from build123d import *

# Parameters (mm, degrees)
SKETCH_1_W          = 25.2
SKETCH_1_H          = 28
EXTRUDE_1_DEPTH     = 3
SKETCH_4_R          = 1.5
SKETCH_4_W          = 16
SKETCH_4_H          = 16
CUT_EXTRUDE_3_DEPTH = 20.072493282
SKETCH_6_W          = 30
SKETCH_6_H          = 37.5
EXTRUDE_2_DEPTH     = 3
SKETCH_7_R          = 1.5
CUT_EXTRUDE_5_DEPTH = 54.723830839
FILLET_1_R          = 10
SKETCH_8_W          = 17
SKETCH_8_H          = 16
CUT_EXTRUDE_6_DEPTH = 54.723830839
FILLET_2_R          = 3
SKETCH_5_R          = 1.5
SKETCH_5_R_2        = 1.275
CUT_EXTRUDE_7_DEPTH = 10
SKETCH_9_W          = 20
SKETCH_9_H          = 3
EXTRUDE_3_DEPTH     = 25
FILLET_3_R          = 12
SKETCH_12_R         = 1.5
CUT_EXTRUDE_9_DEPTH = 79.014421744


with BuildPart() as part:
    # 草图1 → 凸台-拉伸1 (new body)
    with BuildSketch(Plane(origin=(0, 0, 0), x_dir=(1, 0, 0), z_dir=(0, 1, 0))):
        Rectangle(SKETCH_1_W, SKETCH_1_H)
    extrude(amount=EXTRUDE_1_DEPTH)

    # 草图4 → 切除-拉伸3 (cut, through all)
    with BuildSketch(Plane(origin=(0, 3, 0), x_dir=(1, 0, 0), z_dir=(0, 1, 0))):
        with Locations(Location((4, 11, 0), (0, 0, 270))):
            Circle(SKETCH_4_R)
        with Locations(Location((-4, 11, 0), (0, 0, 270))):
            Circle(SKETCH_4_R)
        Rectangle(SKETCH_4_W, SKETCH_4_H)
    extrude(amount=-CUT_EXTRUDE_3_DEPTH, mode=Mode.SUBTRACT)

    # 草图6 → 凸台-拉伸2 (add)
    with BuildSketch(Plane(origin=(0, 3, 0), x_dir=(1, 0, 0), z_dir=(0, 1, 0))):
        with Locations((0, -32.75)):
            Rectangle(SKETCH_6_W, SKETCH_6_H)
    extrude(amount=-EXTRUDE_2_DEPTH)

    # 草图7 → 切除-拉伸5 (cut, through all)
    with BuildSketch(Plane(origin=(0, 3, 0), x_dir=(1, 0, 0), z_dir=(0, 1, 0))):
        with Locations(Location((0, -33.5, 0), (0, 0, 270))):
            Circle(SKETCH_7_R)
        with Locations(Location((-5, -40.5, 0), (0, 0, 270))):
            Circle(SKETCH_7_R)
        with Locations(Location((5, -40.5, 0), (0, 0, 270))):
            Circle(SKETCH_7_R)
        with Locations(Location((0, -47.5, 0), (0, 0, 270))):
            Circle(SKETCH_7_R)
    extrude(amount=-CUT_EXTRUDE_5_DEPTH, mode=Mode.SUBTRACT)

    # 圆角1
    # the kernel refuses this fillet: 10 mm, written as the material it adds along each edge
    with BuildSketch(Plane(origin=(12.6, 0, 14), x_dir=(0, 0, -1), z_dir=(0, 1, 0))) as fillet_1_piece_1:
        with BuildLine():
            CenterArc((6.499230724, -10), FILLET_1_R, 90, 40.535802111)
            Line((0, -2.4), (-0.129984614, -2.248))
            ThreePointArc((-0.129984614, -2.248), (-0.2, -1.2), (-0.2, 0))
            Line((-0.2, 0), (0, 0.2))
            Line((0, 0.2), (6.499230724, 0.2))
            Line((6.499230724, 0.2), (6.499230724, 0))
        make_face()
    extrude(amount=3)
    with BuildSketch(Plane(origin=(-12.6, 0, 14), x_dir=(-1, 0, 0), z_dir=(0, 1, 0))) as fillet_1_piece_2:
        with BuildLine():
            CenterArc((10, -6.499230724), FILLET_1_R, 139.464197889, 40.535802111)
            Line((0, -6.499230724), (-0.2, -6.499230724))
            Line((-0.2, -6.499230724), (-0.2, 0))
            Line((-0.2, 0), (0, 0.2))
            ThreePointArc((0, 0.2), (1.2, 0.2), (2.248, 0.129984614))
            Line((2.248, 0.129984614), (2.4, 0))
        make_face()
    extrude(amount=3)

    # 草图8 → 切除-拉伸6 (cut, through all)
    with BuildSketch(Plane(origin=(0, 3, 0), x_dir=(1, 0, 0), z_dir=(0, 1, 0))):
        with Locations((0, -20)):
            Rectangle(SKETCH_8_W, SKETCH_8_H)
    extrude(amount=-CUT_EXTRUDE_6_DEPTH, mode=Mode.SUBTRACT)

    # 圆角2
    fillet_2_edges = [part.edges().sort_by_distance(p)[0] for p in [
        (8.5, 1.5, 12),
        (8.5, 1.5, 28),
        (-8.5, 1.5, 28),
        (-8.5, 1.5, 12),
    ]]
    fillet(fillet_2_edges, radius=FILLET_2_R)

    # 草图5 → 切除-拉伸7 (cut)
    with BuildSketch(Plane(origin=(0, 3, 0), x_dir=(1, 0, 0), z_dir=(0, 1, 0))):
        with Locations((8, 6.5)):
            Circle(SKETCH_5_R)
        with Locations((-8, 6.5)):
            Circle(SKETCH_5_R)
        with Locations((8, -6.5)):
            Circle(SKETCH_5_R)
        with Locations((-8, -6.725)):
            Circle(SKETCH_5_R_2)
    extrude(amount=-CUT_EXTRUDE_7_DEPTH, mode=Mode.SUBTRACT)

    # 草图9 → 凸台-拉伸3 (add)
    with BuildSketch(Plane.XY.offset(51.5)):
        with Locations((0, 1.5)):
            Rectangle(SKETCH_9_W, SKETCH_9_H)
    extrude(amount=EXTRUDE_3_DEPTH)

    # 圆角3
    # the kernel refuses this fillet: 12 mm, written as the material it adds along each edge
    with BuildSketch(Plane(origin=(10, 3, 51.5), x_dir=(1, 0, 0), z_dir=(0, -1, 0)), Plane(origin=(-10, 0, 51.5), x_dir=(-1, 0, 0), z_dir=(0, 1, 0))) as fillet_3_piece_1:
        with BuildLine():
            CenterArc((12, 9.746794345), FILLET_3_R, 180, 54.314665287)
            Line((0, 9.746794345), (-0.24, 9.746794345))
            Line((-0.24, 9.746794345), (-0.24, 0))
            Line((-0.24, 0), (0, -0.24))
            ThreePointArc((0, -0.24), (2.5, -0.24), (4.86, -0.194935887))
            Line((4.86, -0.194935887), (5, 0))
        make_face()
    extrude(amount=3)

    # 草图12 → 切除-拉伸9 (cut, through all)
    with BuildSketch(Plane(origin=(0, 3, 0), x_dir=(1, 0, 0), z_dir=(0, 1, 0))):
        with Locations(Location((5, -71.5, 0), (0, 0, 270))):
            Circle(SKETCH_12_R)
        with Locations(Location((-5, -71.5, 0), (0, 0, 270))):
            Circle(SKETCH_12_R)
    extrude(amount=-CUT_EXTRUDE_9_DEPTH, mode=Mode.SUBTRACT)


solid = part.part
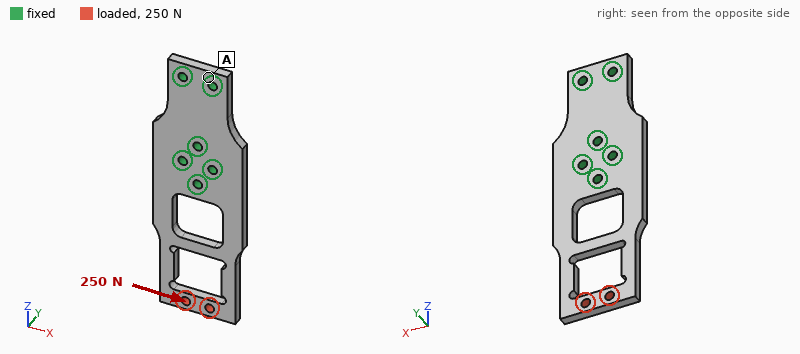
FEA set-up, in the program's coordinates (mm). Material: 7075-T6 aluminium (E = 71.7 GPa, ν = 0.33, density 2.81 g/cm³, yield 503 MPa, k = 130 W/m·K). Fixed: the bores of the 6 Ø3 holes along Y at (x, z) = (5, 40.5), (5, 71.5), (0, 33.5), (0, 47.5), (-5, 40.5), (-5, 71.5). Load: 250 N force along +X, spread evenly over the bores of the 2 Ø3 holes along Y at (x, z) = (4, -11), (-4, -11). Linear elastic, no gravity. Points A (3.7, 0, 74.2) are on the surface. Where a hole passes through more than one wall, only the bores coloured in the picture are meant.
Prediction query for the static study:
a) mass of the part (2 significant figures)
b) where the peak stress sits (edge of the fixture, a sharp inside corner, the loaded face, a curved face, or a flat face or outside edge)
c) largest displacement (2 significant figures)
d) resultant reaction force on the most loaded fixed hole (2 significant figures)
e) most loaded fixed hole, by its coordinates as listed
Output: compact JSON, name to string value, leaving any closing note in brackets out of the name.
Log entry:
{"mass of the part": "15 g", "where the peak stress sits": "a curved face", "largest displacement": "0.22 mm", "resultant reaction force on the most loaded fixed hole": "640 N", "most loaded fixed hole, by its coordinates as listed": "(0, 33.5)"}
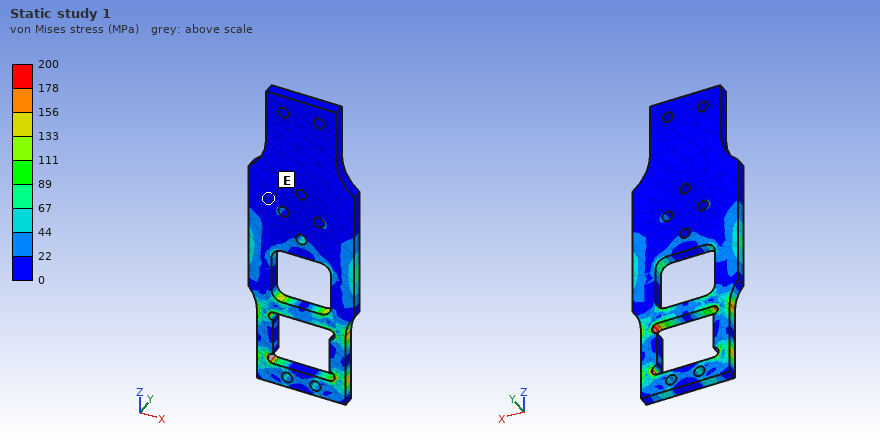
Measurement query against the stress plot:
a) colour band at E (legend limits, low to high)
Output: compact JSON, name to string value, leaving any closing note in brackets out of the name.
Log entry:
{"colour band at E": "0 to 22 MPa"}
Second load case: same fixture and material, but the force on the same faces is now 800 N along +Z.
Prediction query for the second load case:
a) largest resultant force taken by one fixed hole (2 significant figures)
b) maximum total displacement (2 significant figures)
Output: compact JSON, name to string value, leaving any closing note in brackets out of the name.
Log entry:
{"largest resultant force taken by one fixed hole": "280 N", "maximum total displacement": "56 µm"}
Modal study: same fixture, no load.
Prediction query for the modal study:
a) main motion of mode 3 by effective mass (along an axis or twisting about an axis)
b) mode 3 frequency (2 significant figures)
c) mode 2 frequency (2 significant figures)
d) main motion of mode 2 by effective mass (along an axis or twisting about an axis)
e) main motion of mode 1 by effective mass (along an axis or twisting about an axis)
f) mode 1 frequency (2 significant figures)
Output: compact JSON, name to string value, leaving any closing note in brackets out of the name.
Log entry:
{"main motion of mode 3 by effective mass": "along X", "mode 3 frequency": "4000 Hz", "mode 2 frequency": "2900 Hz", "main motion of mode 2 by effective mass": "twisting about Z", "main motion of mode 1 by effective mass": "along Y", "mode 1 frequency": "980 Hz"}
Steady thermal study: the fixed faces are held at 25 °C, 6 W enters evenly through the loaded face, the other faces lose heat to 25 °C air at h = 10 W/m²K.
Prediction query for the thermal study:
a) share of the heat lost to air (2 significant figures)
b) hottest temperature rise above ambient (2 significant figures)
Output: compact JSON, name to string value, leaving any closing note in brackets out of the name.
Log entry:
{"share of the heat lost to air": "12 %", "hottest temperature rise above ambient": "72 K"}
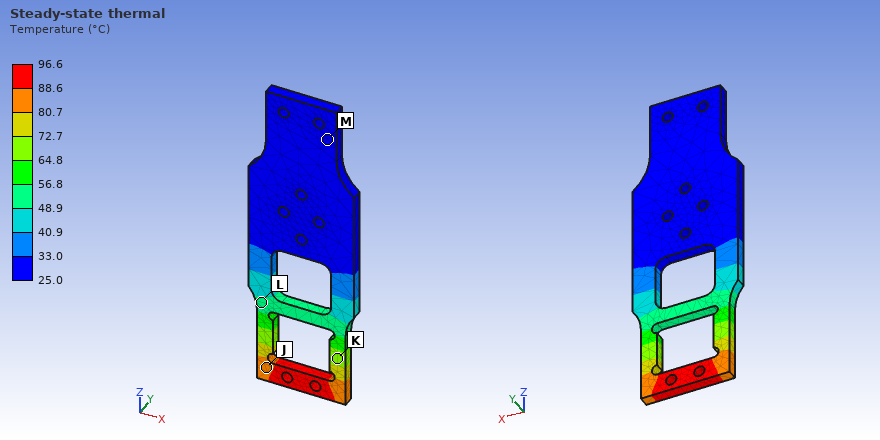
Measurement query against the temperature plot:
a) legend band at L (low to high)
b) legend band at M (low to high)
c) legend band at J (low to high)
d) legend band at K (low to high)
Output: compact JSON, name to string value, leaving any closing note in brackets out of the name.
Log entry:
{"legend band at L": "48.9 to 56.8 °C", "legend band at M": "25.0 to 33.0 °C", "legend band at J": "80.7 to 88.6 °C", "legend band at K": "64.8 to 72.7 °C"}
